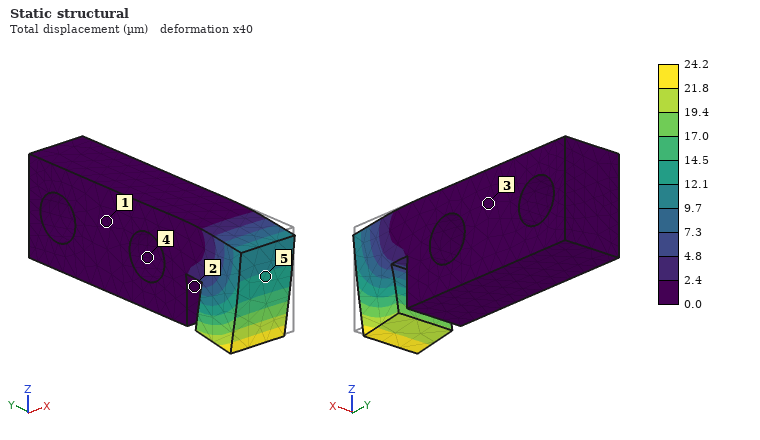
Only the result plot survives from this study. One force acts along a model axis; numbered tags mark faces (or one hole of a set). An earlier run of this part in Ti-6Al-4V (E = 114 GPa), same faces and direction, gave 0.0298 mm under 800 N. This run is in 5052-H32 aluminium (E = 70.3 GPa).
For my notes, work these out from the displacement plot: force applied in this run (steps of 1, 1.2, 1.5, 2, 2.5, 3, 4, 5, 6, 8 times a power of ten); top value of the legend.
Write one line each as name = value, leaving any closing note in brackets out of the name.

force applied in this run = 400 N
top value of the legend = 24.2 µm
